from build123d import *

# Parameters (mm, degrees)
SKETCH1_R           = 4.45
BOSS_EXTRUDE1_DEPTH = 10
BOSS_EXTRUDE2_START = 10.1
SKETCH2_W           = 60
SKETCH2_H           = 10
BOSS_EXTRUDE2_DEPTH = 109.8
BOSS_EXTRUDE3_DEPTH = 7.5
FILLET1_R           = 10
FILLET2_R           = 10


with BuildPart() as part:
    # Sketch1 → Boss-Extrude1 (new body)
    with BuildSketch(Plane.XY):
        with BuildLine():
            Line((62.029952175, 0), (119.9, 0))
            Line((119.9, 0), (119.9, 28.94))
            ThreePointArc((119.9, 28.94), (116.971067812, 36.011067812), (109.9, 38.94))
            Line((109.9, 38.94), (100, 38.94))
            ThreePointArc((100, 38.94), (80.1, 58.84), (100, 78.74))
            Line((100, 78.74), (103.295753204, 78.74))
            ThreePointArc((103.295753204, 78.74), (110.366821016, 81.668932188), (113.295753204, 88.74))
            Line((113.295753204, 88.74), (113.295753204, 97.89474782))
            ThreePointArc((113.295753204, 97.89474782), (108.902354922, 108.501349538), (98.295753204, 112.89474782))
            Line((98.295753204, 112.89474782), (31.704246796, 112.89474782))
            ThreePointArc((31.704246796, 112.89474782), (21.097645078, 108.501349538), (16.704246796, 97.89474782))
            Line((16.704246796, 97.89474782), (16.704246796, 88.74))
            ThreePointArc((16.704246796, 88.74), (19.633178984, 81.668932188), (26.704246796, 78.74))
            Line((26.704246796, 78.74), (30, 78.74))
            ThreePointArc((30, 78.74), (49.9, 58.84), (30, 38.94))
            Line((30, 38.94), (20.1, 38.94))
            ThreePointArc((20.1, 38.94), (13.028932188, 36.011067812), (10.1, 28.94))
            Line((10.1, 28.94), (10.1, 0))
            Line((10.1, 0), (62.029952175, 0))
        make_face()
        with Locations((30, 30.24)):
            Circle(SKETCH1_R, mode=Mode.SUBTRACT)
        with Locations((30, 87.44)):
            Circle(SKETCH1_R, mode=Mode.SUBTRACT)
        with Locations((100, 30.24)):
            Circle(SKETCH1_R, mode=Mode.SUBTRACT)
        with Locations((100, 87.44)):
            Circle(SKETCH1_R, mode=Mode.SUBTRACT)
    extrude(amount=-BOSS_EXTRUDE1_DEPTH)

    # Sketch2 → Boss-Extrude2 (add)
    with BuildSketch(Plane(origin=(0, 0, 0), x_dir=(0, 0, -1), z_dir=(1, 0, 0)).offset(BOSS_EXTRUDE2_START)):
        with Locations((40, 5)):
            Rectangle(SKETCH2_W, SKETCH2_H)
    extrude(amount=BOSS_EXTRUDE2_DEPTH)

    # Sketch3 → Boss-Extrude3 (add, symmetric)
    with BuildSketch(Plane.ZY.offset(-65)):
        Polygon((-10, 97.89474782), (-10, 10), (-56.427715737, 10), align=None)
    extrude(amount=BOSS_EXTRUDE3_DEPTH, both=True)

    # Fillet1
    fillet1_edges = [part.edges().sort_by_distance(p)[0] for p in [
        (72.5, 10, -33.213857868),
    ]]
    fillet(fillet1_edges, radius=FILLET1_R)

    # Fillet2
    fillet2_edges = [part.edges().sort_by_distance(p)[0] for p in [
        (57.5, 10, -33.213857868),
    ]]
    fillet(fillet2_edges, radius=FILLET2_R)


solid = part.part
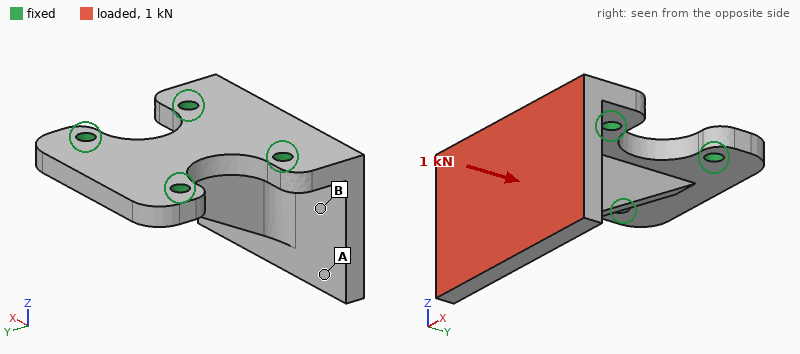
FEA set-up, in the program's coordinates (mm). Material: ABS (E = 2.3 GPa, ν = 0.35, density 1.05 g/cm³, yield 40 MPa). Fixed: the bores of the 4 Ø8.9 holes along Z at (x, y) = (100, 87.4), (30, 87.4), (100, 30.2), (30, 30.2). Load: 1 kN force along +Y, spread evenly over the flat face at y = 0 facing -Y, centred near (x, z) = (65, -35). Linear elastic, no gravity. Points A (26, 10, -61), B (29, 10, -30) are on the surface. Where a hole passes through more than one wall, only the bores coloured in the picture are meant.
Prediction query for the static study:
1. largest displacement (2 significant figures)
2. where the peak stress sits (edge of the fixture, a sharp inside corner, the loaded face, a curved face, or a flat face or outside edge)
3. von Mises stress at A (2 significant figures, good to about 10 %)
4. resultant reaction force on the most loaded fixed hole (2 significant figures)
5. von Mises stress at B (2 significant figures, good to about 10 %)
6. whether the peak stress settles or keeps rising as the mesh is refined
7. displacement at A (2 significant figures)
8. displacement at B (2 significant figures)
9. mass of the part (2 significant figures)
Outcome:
0.71 mm
edge of the fixture
1.1 MPa
350 N
2.3 MPa
keeps rising
0.51 mm
0.24 mm
190 g
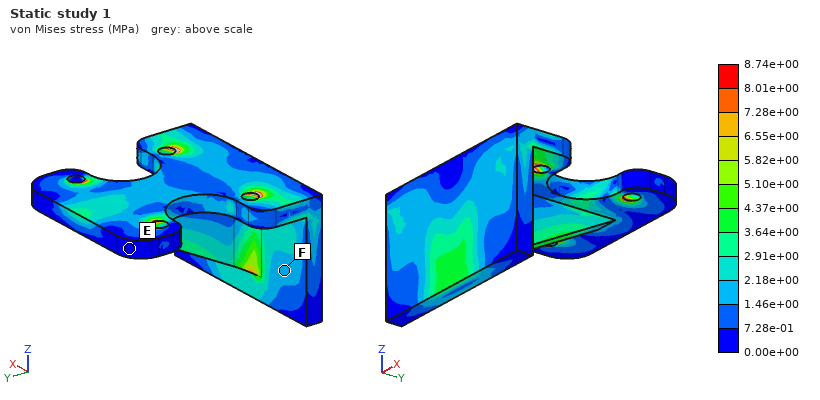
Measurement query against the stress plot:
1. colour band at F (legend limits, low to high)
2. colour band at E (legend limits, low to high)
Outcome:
1.46e+00 to 2.18e+00 MPa
0.00e+00 to 7.28e-01 MPa
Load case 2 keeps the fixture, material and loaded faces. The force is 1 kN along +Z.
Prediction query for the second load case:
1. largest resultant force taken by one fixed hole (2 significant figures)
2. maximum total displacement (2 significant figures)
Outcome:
640 N
0.53 mm
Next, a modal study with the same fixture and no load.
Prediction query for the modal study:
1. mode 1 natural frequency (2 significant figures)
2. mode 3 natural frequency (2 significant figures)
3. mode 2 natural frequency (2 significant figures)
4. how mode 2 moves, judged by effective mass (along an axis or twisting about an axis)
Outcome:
780 Hz
1100 Hz
920 Hz
along X
